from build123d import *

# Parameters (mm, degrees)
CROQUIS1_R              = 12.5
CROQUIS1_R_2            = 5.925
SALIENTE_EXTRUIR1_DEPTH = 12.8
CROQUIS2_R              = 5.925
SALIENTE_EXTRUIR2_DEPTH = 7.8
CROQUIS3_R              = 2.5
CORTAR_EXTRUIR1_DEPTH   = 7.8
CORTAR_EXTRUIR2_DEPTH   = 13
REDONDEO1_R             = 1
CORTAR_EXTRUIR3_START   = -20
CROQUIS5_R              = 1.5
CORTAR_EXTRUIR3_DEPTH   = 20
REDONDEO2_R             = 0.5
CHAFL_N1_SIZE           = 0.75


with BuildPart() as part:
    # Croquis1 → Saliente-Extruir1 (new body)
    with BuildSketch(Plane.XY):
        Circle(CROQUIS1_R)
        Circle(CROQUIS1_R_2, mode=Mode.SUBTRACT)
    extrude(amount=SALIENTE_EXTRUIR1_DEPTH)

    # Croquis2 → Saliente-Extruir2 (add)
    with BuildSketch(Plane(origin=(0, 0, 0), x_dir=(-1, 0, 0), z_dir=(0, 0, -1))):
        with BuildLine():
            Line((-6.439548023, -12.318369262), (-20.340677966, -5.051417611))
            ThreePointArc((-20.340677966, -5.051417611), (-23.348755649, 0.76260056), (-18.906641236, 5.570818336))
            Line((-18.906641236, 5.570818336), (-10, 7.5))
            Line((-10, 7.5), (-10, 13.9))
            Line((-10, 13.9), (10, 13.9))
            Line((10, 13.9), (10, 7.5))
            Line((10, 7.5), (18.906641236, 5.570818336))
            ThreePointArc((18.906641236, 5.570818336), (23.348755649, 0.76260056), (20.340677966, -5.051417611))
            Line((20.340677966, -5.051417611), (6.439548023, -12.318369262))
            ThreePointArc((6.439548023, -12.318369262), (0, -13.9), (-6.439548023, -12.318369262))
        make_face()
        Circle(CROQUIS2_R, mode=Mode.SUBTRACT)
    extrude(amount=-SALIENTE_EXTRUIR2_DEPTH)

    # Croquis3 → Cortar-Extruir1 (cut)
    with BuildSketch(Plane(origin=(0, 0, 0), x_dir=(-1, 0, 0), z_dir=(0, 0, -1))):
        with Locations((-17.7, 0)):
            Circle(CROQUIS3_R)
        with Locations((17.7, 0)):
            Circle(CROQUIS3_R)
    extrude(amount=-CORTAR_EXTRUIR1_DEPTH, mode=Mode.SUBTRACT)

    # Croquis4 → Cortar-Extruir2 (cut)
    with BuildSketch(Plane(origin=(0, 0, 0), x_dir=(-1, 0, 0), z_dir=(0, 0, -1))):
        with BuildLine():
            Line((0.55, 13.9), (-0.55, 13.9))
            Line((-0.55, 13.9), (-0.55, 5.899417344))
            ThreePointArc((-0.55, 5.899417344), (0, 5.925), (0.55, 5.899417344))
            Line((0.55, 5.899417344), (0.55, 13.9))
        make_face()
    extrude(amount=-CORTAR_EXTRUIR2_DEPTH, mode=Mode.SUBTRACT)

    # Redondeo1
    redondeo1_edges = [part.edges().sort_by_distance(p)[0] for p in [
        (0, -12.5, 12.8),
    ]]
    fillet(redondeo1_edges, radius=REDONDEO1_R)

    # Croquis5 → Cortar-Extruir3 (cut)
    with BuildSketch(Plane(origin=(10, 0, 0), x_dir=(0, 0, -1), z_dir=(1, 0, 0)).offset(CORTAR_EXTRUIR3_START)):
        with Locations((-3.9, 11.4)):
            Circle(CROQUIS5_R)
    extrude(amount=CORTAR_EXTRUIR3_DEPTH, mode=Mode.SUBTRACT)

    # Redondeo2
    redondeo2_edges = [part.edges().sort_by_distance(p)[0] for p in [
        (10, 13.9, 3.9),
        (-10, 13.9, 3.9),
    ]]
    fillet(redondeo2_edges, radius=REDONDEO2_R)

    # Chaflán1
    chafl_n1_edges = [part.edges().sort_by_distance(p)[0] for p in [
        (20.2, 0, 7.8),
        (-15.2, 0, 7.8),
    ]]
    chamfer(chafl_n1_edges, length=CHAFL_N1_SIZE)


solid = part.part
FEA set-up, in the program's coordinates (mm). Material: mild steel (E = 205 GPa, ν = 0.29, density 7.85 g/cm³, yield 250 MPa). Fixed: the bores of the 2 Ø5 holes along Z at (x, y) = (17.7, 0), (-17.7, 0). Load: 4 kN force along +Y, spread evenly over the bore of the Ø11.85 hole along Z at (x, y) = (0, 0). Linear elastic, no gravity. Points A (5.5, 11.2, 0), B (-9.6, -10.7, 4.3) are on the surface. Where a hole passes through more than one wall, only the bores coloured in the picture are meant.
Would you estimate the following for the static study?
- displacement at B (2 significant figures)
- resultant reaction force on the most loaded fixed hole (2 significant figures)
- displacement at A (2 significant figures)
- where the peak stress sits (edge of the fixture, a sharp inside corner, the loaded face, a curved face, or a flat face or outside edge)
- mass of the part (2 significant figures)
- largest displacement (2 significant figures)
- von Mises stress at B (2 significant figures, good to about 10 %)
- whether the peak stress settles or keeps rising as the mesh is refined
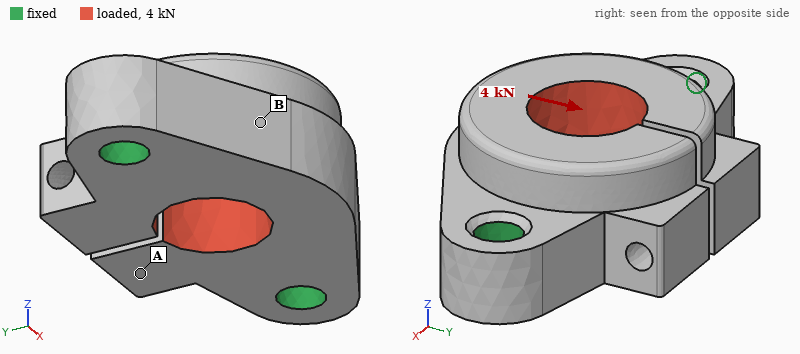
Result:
4.7 µm
2.6 kN
7.6 µm
edge of the fixture
57 g
14 µm
46 MPa
keeps rising
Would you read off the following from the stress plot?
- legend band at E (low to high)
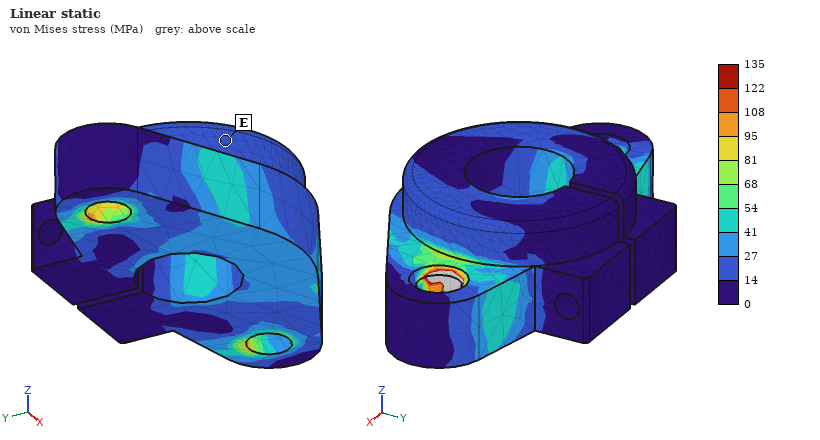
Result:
14 to 27 MPa
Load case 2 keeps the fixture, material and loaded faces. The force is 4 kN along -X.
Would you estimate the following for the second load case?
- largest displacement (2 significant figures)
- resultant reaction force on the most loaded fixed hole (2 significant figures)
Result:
4.1 µm
2.0 kN
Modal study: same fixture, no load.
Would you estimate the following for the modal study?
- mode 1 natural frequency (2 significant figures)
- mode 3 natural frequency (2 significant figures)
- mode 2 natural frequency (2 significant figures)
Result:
15 kHz
17 kHz
17 kHz
